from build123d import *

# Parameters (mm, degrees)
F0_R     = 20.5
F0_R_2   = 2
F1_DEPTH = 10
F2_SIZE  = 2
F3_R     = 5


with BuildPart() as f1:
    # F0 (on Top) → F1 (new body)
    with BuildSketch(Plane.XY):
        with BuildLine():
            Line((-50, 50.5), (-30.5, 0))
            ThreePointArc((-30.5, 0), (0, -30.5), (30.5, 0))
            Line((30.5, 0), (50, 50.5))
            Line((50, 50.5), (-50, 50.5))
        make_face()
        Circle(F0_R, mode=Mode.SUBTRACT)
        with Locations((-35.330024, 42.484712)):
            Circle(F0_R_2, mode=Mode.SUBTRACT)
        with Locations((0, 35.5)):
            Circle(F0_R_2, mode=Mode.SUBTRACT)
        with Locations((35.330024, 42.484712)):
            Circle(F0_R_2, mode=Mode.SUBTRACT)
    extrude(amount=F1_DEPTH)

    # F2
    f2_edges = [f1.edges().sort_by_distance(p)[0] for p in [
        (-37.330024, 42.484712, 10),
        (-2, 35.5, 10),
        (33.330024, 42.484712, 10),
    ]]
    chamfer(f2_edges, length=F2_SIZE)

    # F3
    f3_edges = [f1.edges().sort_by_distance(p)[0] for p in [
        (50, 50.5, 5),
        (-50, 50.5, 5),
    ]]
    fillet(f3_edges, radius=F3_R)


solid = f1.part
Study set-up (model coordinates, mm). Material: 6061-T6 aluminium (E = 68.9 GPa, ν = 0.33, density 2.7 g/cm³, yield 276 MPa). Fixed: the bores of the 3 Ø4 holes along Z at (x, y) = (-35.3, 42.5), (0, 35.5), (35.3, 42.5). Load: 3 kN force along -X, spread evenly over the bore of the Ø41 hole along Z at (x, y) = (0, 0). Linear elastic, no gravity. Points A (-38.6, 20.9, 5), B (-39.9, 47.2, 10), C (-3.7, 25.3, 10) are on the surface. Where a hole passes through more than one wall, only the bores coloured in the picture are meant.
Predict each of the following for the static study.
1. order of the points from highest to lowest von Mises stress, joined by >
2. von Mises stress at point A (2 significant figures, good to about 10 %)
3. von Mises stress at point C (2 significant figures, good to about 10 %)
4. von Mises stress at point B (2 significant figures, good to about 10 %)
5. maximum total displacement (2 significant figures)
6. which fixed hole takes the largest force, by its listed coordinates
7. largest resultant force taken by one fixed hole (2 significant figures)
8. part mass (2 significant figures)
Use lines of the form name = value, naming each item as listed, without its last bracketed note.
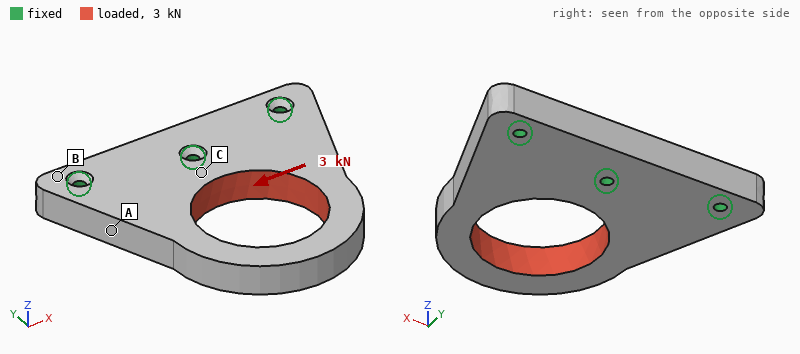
order of the points from highest to lowest von Mises stress, joined by > = A > C > B
von Mises stress at point A = 19 MPa
von Mises stress at point C = 13 MPa
von Mises stress at point B = 5.0 MPa
maximum total displacement = 46 µm
which fixed hole takes the largest force, by its listed coordinates = (0, 35.5)
largest resultant force taken by one fixed hole = 1.9 kN
part mass = 110 g
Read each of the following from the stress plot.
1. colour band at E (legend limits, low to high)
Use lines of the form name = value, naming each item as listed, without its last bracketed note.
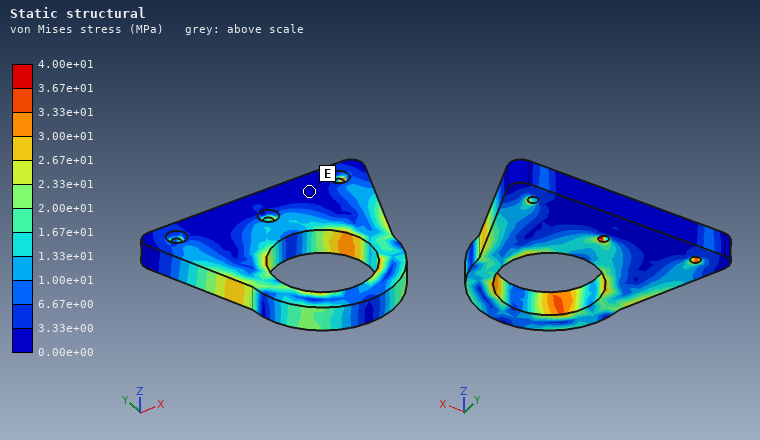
colour band at E = 0.00e+00 to 3.33e+00 MPa
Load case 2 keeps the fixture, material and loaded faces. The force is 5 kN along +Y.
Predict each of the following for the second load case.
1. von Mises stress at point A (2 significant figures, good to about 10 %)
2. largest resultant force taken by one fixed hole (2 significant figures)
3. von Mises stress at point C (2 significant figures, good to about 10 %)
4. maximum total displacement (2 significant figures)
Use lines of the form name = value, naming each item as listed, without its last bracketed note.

von Mises stress at point A = 11 MPa
largest resultant force taken by one fixed hole = 1.7 kN
von Mises stress at point C = 5.8 MPa
maximum total displacement = 20 µm
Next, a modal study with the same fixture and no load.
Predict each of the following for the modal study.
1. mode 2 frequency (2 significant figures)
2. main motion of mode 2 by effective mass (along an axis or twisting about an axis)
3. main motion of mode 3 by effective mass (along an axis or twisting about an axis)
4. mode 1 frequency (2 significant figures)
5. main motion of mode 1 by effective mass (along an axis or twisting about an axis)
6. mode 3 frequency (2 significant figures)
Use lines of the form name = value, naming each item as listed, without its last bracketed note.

mode 2 frequency = 4600 Hz
main motion of mode 2 by effective mass = twisting about Y
main motion of mode 3 by effective mass = along X
mode 1 frequency = 2000 Hz
main motion of mode 1 by effective mass = along Z
mode 3 frequency = 6800 Hz
